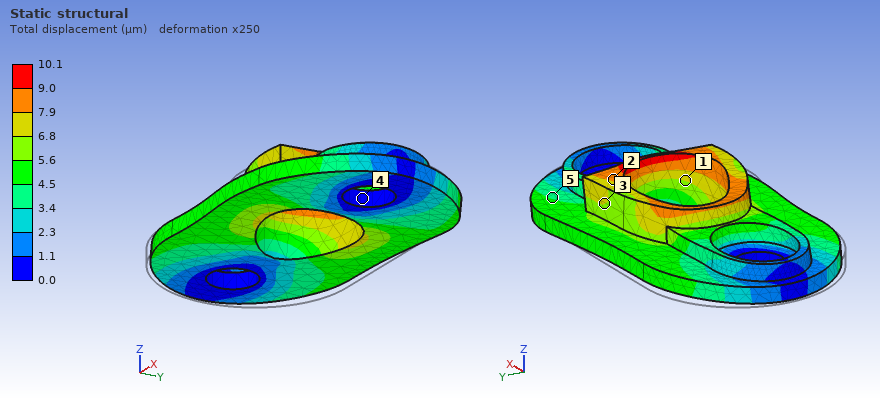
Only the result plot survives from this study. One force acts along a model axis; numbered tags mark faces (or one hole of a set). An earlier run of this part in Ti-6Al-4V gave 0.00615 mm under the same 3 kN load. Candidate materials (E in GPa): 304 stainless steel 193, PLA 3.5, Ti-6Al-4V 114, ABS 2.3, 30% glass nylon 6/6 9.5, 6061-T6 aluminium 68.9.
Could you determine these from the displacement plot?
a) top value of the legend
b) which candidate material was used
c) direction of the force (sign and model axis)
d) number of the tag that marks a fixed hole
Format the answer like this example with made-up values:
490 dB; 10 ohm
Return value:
10.1 µm; 6061-T6 aluminium; +X; 4
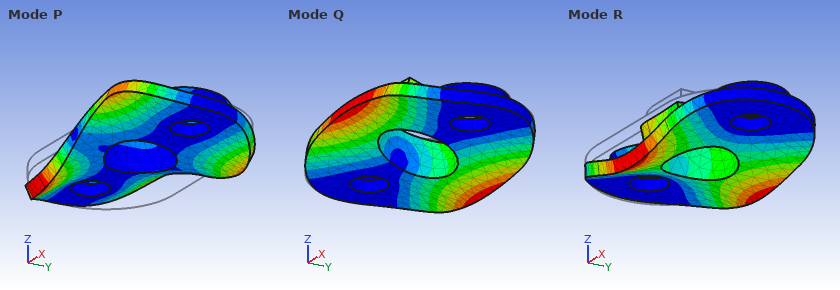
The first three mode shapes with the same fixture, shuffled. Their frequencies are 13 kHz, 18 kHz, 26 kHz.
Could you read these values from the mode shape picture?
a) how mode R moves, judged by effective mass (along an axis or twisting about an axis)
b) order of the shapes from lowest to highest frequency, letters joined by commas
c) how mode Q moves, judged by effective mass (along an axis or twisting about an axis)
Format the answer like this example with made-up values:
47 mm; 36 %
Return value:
along Z; Q, R, P; twisting about X
